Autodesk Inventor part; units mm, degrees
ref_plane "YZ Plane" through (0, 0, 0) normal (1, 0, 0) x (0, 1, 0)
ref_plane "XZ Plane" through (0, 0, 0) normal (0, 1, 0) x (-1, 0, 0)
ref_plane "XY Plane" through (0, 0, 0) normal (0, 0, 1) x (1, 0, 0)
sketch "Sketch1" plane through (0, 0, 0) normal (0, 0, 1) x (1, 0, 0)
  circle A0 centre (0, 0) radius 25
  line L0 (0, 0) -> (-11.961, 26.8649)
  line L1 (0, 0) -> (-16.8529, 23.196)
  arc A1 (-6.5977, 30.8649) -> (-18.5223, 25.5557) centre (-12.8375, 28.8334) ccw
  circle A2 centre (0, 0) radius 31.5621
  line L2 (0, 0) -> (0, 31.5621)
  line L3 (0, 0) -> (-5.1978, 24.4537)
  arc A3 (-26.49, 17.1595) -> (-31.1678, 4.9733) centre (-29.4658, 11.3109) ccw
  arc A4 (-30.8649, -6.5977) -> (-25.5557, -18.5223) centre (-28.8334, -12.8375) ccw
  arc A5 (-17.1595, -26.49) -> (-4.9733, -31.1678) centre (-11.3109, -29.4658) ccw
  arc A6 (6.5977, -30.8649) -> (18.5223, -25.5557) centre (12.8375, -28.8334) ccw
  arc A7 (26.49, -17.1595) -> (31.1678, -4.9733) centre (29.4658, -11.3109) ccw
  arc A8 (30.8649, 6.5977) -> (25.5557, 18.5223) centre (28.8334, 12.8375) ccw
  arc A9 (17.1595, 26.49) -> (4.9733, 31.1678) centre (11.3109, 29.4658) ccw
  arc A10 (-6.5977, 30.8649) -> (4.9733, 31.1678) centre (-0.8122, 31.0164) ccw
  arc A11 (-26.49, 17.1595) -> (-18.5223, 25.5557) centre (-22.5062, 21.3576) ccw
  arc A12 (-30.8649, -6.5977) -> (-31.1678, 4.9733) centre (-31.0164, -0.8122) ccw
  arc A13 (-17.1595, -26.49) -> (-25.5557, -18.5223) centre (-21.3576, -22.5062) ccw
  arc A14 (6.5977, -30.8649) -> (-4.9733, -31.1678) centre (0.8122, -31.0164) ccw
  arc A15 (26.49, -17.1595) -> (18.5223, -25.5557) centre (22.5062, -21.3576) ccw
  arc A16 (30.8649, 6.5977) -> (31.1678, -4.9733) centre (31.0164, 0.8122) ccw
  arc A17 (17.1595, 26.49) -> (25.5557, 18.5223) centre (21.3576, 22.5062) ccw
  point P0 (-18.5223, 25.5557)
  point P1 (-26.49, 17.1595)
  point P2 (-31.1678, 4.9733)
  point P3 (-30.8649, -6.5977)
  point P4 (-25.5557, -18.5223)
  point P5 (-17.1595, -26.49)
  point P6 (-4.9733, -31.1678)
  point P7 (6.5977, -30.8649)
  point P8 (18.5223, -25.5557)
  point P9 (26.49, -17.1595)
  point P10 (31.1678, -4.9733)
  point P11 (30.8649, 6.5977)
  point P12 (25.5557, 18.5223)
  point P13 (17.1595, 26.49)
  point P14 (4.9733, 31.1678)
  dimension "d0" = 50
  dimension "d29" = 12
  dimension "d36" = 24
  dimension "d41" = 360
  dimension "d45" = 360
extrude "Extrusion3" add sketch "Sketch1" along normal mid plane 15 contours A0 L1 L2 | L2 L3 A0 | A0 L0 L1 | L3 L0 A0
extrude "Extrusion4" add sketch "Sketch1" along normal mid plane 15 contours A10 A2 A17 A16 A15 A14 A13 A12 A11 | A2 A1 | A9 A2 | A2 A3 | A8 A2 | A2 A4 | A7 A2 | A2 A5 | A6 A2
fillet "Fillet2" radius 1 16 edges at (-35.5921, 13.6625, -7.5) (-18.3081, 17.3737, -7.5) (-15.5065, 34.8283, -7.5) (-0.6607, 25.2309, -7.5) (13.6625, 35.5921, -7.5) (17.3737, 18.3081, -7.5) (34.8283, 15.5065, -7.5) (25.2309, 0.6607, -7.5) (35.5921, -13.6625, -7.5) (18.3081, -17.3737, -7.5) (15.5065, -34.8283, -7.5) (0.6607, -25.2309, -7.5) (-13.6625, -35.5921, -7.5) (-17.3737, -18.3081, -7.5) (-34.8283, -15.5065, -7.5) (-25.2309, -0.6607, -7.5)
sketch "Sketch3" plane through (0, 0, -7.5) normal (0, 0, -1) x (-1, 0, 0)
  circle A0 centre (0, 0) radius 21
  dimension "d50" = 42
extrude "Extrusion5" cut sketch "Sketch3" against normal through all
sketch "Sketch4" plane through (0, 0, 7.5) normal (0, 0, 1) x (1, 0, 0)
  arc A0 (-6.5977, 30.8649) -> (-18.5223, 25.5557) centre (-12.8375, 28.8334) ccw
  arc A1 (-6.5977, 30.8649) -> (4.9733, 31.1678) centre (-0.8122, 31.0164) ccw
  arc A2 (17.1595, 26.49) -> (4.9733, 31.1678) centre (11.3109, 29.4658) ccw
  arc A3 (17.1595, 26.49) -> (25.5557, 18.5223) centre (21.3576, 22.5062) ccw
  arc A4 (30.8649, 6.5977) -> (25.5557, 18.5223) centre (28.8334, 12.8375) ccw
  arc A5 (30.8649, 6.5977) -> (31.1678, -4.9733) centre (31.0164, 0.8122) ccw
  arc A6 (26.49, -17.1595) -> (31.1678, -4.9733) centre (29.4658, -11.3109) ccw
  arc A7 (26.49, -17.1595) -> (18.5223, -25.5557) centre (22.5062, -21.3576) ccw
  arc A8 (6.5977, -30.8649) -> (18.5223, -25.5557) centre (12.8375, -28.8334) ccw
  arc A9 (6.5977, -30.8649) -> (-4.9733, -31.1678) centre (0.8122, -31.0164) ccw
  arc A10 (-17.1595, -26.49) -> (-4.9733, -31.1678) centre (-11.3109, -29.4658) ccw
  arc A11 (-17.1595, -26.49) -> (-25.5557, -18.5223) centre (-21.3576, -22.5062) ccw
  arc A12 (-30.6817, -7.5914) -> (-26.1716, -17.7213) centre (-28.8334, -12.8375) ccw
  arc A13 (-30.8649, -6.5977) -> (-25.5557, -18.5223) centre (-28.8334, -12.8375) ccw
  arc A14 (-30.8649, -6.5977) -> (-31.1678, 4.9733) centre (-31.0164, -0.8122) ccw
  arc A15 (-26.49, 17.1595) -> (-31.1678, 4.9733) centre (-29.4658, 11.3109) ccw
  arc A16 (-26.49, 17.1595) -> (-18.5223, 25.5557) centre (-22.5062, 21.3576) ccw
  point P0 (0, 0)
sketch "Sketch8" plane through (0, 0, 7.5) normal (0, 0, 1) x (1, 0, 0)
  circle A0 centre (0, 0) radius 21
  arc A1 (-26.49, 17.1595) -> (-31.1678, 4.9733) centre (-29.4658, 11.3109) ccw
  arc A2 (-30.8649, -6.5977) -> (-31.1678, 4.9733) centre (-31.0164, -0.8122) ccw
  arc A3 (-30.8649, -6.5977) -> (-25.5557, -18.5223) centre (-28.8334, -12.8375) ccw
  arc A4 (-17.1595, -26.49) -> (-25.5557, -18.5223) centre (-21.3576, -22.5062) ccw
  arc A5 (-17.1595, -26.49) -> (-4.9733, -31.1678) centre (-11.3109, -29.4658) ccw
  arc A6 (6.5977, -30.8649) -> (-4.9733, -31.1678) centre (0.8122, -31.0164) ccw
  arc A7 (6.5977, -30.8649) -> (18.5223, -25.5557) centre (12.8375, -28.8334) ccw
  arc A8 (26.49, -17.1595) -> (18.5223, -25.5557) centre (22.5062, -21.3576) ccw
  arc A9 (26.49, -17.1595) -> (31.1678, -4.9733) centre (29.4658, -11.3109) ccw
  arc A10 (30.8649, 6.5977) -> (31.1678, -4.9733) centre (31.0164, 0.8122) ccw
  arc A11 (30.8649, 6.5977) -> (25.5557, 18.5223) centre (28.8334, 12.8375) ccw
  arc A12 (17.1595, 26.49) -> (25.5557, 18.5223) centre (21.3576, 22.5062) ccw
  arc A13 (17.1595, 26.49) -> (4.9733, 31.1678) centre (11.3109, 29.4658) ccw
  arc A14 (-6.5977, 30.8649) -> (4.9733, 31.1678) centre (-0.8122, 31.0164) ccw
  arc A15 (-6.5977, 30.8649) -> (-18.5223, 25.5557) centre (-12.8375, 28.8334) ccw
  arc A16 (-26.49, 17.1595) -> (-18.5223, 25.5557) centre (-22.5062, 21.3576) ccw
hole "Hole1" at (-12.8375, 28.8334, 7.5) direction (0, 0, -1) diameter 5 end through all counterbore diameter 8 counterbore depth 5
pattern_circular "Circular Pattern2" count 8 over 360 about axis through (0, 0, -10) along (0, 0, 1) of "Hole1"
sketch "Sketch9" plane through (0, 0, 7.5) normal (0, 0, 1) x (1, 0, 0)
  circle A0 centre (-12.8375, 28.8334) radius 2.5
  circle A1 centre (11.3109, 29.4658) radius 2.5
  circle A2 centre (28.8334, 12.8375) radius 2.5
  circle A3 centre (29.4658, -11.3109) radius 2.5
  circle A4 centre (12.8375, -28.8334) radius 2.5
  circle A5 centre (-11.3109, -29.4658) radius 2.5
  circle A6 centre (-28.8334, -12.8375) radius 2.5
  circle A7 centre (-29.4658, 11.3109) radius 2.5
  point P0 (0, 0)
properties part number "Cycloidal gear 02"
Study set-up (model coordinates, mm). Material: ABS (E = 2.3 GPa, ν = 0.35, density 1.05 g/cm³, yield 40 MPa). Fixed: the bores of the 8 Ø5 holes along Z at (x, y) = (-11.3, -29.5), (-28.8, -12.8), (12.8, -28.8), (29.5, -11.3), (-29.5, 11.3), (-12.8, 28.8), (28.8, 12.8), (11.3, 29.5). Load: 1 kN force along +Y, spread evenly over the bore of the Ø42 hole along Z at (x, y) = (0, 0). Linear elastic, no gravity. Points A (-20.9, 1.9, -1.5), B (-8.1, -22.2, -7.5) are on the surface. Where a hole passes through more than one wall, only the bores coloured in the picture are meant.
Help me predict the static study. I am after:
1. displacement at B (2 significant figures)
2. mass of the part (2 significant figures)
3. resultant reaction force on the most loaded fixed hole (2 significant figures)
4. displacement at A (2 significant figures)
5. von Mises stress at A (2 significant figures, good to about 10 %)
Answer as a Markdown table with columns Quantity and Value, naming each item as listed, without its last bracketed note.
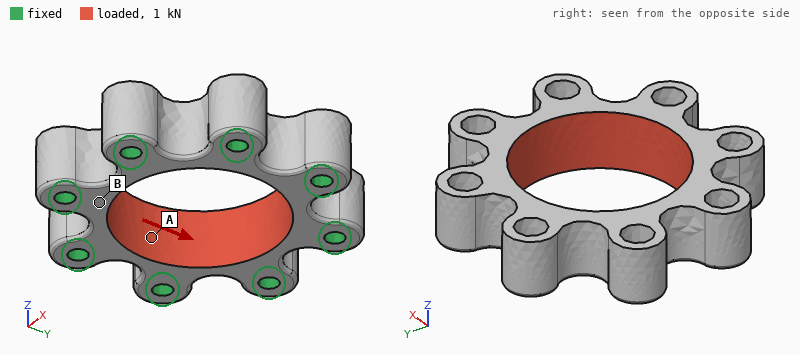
| Quantity | Value |
|---|---|
| displacement at B | 2.6 µm |
| mass of the part | 25 g |
| resultant reaction force on the most loaded fixed hole | 170 N |
| displacement at A | 6.3 µm |
| von Mises stress at A | 1.2 MPa |
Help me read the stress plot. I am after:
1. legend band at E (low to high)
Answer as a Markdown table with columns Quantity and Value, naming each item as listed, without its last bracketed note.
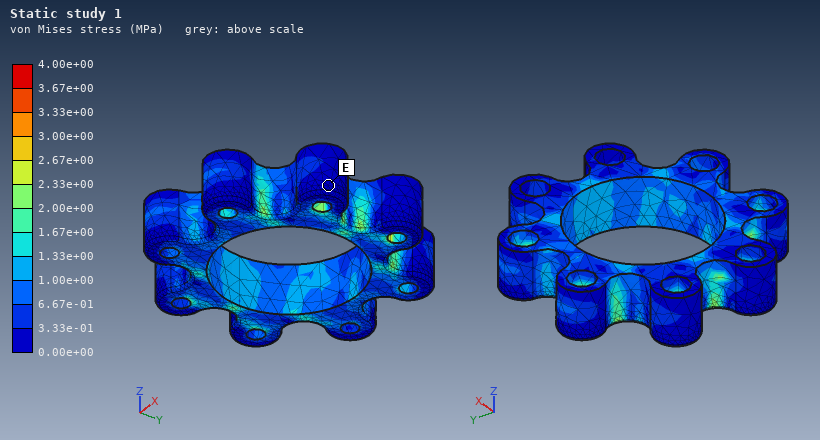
| Quantity | Value |
|---|---|
| legend band at E | 0.00e+00 to 3.33e-01 MPa |
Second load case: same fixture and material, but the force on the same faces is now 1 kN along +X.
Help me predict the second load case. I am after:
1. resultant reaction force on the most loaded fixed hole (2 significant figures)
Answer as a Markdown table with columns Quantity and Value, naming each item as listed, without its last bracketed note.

| Quantity | Value |
|---|---|
| resultant reaction force on the most loaded fixed hole | 170 N |
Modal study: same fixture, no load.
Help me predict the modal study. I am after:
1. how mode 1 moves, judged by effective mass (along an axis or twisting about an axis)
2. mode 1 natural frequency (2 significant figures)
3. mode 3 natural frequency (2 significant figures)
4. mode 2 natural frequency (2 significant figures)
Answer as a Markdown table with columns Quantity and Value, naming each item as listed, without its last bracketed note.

| Quantity | Value |
|---|---|
| how mode 1 moves, judged by effective mass | along Z |
| mode 1 natural frequency | 11 kHz |
| mode 3 natural frequency | 12 kHz |
| mode 2 natural frequency | 12 kHz |
